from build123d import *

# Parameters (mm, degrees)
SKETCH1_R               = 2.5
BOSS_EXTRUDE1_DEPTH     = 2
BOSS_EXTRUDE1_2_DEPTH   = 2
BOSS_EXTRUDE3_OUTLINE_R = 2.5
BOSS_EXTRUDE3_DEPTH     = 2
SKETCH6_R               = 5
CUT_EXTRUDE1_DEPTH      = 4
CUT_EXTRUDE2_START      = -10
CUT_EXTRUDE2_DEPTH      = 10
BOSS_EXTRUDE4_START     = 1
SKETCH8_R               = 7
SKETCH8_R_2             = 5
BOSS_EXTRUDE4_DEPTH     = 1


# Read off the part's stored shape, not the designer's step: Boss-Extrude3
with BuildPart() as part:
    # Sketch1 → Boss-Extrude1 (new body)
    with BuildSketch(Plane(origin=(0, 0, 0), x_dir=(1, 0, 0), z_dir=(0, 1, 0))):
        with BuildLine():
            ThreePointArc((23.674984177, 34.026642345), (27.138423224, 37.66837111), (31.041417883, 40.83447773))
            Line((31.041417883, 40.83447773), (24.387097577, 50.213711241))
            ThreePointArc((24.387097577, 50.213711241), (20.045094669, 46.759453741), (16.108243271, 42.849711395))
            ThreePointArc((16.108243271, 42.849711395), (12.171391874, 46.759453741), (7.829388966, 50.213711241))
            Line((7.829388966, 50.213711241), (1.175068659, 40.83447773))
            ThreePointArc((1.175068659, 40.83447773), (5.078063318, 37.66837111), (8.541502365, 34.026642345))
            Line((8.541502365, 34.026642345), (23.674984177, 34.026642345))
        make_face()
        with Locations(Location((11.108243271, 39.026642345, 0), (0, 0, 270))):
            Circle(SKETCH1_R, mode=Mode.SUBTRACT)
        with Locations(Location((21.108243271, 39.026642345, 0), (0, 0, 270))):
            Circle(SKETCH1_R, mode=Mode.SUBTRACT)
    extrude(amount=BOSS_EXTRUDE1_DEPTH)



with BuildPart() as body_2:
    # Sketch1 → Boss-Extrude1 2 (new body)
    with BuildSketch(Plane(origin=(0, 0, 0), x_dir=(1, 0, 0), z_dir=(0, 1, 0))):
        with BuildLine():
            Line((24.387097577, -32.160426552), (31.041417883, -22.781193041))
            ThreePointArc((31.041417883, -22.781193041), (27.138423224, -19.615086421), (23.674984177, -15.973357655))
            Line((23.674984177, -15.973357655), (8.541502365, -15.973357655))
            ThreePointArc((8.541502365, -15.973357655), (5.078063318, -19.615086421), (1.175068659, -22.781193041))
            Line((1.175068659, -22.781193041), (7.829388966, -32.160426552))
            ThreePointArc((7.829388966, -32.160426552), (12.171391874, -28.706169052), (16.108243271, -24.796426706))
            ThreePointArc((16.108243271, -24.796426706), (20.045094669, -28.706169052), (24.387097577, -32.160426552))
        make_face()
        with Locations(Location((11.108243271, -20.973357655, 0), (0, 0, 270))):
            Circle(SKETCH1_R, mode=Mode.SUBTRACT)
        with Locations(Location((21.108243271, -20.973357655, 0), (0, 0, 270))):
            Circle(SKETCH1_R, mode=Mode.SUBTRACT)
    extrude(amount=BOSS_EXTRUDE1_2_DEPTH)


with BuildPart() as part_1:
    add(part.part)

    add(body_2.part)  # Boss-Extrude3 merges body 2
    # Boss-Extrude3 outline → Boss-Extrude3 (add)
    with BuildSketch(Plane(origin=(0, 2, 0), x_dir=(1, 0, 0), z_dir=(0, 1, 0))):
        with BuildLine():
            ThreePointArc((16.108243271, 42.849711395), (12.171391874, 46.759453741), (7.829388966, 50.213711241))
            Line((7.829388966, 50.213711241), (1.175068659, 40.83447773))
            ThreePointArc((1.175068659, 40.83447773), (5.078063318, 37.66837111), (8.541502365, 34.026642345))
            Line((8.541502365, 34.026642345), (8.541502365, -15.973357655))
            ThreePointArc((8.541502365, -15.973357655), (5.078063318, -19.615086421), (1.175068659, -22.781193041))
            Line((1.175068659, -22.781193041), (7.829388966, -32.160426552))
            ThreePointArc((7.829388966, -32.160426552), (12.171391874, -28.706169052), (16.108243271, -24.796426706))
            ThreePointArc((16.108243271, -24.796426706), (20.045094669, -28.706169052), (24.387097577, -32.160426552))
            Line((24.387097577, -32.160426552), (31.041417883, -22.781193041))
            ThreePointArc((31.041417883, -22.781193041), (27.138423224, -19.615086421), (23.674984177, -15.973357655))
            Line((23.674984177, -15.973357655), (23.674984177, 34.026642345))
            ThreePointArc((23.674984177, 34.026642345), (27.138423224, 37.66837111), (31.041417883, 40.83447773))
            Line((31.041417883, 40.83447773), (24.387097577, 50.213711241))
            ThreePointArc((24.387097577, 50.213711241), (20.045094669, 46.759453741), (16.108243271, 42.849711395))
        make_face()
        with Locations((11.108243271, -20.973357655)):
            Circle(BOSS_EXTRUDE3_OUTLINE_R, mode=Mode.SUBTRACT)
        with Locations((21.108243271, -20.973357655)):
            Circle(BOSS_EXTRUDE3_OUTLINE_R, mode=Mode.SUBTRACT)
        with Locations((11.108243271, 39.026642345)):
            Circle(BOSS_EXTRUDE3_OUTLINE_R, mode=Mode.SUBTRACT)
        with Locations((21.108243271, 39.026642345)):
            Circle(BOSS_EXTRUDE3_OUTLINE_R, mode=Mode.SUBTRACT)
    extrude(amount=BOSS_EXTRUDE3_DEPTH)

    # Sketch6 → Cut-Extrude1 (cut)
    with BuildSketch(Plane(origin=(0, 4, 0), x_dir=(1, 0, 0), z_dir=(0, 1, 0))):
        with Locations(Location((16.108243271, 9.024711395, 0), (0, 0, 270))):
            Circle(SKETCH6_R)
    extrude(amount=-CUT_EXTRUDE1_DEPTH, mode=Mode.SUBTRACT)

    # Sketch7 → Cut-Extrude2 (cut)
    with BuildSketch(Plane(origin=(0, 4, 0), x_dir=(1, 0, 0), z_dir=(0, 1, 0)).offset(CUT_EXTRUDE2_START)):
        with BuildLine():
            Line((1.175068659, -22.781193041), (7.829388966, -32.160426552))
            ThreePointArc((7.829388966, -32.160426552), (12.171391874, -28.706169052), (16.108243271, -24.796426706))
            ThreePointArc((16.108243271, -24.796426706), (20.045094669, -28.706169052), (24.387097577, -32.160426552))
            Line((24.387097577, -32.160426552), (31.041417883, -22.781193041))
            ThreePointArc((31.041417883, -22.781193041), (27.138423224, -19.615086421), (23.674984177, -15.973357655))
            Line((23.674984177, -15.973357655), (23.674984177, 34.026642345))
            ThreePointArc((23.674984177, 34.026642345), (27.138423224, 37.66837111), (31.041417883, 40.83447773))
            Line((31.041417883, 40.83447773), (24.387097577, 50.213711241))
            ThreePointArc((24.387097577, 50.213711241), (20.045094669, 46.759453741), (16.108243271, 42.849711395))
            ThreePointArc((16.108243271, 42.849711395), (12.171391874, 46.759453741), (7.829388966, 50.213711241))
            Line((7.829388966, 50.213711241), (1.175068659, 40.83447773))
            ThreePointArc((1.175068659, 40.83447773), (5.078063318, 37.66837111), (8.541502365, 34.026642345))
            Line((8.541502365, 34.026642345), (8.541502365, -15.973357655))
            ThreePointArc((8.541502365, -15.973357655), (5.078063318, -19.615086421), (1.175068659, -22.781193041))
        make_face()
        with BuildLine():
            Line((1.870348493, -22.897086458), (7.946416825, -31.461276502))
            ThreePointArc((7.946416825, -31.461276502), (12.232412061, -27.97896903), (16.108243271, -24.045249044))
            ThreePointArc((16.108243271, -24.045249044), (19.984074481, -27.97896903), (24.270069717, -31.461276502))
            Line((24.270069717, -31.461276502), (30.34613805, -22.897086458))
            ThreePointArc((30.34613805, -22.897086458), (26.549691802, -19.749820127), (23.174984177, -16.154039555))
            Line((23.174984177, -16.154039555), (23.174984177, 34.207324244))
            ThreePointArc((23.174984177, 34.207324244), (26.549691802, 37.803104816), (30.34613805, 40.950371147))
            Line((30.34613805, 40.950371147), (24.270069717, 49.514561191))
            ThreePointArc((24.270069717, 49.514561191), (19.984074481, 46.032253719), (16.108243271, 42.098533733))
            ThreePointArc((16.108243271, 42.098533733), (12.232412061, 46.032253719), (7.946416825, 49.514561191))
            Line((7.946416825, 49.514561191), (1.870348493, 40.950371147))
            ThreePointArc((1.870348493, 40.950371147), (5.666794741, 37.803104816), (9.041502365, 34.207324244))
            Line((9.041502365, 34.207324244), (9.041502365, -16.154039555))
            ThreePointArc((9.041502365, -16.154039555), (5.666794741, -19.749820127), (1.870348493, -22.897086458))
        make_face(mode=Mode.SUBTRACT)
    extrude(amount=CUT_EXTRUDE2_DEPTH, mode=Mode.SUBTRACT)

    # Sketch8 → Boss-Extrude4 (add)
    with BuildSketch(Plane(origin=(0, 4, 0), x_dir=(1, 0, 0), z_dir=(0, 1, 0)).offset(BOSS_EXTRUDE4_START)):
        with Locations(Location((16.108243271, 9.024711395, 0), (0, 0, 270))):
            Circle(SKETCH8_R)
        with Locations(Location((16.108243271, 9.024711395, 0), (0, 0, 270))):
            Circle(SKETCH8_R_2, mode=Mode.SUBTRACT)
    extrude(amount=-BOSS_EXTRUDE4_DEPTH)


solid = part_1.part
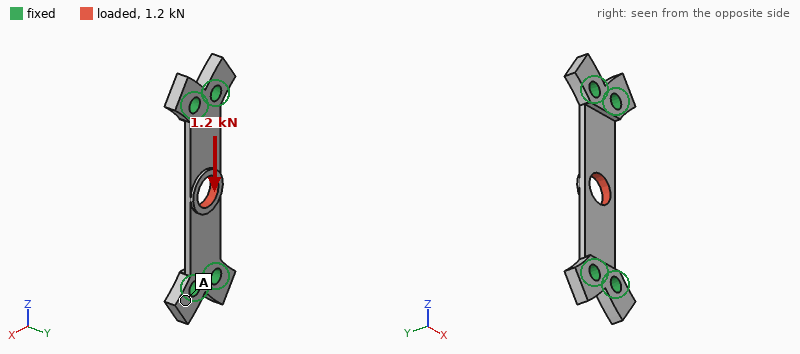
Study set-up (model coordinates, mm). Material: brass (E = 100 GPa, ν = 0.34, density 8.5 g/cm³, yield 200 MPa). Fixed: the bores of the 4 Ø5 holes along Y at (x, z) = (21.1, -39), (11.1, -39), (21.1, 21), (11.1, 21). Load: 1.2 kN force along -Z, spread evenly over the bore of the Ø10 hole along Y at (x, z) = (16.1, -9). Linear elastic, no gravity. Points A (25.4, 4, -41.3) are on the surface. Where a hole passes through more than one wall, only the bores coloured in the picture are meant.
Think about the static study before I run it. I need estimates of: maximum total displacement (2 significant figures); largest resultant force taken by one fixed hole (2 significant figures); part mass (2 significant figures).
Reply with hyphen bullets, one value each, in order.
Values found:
- 7.1 µm
- 310 N
- 28 g
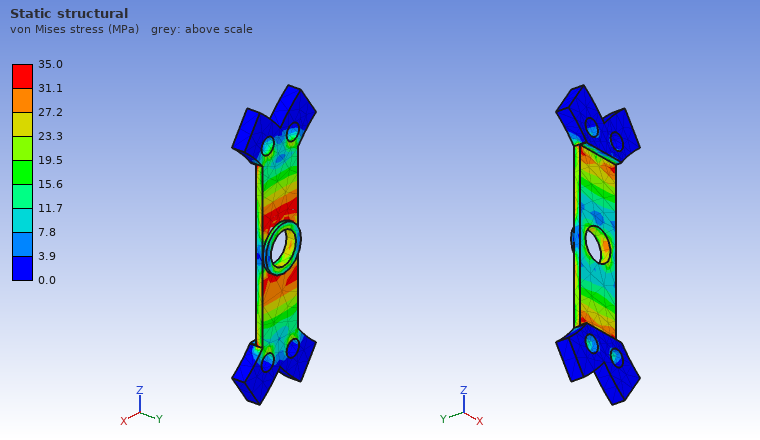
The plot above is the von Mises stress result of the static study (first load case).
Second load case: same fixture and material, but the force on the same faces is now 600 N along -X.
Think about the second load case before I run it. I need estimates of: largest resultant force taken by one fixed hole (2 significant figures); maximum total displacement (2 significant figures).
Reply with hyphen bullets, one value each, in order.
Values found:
- 420 N
- 25 µm
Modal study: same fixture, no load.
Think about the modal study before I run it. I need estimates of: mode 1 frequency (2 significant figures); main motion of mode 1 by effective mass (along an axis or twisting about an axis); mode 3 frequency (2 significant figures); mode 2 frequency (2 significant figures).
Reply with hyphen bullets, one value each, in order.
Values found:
- 2800 Hz
- along Y
- 7000 Hz
- 6200 Hz
